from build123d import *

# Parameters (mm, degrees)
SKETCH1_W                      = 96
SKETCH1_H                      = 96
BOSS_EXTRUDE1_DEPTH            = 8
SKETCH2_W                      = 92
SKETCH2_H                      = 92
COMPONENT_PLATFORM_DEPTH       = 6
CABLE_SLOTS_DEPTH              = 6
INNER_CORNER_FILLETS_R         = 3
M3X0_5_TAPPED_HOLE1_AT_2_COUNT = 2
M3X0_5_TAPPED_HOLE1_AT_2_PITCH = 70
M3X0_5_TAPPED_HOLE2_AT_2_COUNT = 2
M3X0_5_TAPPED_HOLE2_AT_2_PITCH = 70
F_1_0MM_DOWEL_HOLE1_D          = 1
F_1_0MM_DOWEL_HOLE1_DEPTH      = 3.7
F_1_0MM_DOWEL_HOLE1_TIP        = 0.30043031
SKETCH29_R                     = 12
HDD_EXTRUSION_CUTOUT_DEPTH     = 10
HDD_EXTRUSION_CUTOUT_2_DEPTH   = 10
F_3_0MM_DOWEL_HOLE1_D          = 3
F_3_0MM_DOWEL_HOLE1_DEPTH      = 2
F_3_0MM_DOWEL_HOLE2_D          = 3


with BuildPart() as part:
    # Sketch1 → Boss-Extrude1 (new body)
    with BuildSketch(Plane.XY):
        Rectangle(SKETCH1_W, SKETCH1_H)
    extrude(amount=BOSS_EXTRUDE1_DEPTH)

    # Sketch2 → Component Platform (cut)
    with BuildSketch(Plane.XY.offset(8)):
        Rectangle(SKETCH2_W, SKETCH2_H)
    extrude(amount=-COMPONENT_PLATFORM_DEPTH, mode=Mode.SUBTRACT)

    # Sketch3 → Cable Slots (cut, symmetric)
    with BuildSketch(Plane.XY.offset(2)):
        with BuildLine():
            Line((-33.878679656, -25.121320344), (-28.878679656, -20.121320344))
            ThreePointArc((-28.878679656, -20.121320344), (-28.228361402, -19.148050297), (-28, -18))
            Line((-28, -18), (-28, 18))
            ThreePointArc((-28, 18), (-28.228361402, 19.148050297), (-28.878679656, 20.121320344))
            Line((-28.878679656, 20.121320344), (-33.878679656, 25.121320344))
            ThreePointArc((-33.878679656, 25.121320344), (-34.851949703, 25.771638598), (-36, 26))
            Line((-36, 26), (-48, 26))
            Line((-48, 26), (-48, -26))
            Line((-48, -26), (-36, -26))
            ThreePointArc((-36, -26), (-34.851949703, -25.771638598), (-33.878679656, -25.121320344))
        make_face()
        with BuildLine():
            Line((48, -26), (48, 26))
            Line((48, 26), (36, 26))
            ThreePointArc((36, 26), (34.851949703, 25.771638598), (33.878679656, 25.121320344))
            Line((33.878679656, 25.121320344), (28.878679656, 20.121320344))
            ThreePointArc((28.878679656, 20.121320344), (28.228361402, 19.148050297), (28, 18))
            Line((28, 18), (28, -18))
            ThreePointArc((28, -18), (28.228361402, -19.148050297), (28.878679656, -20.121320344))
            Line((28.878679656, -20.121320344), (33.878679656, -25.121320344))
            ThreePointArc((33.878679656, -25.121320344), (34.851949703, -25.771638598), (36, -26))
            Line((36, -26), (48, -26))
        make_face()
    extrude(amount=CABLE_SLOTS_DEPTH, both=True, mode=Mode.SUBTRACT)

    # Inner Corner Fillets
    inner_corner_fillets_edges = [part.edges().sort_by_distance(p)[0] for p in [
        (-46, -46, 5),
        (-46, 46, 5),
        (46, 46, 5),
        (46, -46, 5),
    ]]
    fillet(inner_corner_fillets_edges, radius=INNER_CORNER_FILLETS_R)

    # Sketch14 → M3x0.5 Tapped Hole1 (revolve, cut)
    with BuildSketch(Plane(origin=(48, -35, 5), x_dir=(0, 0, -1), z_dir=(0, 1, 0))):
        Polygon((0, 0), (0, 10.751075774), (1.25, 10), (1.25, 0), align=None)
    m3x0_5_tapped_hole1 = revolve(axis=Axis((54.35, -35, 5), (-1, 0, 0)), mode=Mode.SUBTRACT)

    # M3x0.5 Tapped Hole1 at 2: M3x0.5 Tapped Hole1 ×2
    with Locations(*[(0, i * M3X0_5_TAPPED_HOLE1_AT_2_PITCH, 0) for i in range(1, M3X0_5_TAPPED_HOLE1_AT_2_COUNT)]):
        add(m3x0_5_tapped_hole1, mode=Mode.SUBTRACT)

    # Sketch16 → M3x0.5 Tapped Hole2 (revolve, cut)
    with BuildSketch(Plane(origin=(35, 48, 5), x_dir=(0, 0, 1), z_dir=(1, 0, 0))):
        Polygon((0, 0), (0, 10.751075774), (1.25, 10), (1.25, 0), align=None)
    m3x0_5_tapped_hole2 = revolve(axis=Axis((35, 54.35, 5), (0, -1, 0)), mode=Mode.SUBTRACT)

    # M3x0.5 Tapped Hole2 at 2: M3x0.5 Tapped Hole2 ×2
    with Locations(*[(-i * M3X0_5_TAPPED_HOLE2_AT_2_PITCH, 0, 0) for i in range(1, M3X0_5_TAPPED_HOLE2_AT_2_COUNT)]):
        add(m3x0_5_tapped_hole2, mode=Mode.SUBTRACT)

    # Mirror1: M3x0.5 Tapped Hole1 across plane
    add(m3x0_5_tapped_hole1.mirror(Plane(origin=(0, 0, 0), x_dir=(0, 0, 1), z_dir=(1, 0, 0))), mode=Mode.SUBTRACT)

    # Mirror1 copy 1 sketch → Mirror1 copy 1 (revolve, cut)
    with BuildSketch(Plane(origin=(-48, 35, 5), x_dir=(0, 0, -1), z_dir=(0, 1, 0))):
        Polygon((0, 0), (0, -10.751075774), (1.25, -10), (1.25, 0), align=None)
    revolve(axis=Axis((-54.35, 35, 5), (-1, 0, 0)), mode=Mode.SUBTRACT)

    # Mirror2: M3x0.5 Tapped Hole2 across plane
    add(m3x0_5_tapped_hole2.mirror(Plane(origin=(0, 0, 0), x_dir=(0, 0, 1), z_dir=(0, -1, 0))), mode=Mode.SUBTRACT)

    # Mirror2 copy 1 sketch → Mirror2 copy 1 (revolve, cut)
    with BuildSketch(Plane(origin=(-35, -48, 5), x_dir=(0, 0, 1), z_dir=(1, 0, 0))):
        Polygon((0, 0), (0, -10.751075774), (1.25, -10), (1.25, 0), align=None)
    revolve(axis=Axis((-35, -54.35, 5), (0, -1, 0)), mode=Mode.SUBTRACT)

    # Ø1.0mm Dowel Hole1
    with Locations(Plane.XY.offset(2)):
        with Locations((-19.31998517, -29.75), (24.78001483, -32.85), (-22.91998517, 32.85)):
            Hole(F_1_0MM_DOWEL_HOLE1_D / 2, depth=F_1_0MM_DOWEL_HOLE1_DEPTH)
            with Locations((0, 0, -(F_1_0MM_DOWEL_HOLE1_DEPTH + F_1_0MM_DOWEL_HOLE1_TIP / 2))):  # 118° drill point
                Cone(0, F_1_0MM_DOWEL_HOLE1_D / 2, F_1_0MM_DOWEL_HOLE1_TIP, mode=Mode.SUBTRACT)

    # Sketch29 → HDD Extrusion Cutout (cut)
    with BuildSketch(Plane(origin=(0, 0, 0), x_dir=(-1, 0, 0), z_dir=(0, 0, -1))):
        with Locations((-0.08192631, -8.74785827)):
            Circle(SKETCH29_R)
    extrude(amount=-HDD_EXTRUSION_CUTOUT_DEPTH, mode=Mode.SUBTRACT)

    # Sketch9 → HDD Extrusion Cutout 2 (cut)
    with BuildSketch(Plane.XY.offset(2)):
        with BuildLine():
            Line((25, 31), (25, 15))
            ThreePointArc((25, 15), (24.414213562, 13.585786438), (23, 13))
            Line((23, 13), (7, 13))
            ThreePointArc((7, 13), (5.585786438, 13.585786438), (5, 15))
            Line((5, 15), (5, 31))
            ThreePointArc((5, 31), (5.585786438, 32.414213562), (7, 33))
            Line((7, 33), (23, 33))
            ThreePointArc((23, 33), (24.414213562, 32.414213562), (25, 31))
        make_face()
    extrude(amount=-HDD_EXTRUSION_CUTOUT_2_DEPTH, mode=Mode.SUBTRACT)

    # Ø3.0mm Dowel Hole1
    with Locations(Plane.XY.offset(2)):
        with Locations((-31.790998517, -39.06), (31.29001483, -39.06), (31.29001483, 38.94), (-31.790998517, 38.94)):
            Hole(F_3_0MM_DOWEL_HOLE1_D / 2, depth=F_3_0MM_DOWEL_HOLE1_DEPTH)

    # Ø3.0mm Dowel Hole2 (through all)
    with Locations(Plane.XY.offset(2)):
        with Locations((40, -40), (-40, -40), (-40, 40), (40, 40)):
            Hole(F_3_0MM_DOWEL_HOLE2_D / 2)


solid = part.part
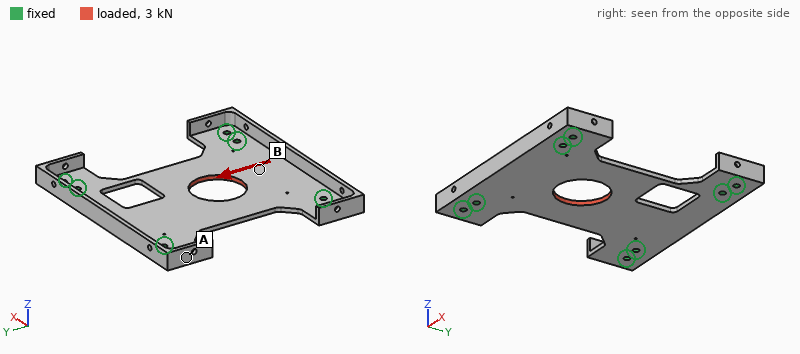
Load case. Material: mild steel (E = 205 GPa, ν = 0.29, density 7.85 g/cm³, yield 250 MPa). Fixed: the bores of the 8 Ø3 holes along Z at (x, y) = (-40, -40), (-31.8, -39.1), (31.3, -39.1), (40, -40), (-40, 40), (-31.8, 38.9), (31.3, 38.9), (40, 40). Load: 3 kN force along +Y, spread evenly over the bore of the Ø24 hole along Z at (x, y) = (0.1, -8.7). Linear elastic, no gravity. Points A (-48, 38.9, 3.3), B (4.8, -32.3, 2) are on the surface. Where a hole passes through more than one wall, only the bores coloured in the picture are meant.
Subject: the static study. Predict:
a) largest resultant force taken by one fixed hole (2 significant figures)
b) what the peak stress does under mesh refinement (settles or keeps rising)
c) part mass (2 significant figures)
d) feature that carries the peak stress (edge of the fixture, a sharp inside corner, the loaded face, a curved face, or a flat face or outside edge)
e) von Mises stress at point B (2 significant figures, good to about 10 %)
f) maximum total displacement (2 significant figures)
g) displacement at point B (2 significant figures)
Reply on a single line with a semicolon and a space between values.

1.0 kN; keeps rising; 120 g; edge of the fixture; 11 MPa; 9.6 µm; 7.3 µm
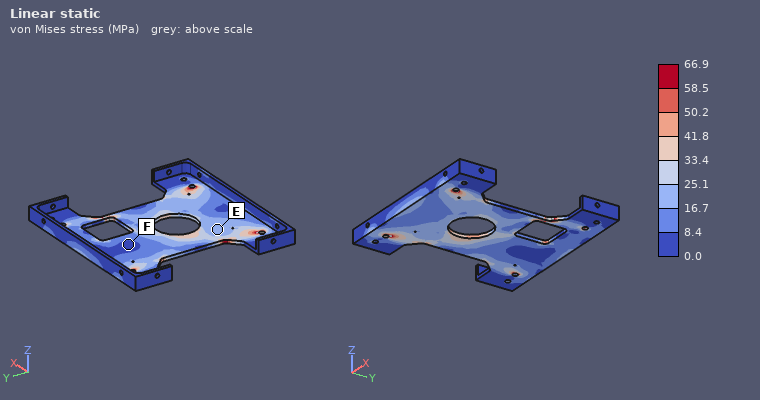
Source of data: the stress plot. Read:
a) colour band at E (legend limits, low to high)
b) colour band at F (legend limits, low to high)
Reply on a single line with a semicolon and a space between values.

16.7 to 25.1 MPa; 0.0 to 8.4 MPa
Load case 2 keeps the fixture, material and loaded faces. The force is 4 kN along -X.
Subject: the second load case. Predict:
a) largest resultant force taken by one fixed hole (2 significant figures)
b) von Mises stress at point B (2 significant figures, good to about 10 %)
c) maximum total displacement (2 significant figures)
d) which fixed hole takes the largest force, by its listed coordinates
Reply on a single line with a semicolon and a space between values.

1.0 kN; 35 MPa; 15 µm; (-31.8, -39.1)
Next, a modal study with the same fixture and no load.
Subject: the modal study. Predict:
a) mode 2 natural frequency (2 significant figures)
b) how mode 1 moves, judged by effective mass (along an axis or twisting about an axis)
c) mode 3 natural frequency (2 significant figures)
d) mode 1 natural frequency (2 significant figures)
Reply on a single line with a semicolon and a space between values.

2500 Hz; along Z; 3200 Hz; 1500 Hz
